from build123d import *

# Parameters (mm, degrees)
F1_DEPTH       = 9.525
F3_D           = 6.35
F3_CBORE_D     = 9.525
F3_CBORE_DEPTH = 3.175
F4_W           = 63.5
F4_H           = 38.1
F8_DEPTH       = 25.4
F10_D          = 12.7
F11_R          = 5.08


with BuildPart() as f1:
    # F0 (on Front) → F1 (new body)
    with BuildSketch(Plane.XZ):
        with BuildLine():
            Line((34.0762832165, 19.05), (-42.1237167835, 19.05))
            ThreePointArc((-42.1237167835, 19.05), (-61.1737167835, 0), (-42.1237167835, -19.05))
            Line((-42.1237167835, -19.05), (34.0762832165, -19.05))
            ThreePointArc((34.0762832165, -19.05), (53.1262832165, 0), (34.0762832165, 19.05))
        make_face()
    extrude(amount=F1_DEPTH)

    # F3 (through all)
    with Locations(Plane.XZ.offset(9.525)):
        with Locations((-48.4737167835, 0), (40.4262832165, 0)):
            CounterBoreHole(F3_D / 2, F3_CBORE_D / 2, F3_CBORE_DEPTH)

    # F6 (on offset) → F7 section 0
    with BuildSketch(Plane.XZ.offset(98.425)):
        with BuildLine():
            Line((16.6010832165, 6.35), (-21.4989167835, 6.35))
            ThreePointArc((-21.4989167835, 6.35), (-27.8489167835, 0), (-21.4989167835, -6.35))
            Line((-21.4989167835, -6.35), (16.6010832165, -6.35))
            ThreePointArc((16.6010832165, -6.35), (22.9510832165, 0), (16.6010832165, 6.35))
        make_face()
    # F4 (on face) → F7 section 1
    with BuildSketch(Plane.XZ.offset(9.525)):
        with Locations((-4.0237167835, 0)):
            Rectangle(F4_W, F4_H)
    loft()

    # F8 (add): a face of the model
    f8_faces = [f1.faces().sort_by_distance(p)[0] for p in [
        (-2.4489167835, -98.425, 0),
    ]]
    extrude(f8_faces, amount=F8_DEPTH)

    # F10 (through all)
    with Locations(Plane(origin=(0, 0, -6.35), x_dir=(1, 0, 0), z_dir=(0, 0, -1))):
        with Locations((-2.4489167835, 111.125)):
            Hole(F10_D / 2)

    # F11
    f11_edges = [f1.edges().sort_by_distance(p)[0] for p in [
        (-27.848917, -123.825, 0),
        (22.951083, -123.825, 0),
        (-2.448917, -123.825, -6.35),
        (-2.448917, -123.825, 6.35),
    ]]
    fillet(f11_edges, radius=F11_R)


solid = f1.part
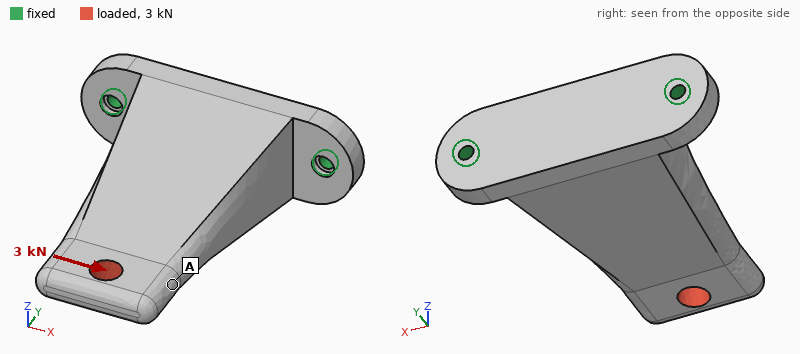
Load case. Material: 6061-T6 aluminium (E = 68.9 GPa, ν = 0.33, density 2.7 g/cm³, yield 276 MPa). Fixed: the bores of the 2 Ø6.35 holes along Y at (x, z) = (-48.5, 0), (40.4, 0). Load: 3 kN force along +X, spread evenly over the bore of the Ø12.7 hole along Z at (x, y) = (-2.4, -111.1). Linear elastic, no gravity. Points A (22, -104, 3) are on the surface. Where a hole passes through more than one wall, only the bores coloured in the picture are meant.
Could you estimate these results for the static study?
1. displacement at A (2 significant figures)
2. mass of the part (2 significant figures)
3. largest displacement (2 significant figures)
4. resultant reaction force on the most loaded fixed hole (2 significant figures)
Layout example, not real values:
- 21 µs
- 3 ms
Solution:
- 0.12 mm
- 480 g
- 0.15 mm
- 4.3 kN
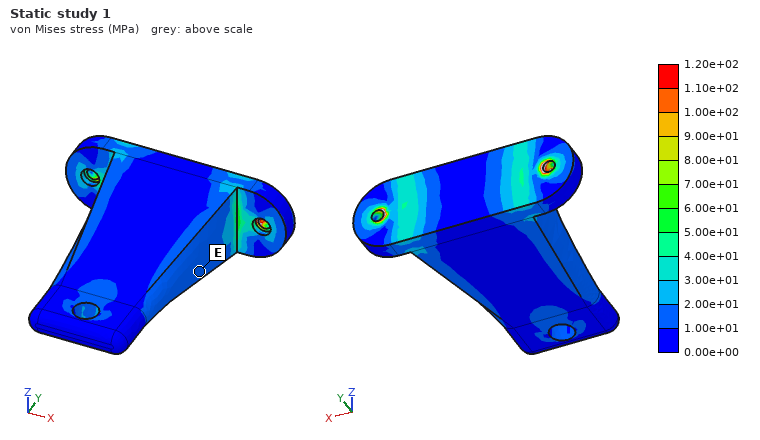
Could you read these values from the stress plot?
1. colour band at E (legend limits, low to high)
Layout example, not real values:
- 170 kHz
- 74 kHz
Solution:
- 1.00e+01 to 2.00e+01 MPa
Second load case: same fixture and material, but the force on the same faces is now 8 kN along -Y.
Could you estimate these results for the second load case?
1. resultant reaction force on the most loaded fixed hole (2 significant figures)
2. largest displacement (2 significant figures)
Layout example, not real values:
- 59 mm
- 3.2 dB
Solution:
- 5.0 kN
- 51 µm
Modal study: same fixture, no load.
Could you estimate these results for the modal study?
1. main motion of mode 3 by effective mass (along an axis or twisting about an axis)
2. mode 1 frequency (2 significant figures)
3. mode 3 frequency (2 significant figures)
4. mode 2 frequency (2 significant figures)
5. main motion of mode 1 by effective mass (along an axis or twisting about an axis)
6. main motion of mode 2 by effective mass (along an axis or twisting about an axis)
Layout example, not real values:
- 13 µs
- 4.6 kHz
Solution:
- along Y
- 640 Hz
- 3800 Hz
- 2500 Hz
- along Z
- along X
